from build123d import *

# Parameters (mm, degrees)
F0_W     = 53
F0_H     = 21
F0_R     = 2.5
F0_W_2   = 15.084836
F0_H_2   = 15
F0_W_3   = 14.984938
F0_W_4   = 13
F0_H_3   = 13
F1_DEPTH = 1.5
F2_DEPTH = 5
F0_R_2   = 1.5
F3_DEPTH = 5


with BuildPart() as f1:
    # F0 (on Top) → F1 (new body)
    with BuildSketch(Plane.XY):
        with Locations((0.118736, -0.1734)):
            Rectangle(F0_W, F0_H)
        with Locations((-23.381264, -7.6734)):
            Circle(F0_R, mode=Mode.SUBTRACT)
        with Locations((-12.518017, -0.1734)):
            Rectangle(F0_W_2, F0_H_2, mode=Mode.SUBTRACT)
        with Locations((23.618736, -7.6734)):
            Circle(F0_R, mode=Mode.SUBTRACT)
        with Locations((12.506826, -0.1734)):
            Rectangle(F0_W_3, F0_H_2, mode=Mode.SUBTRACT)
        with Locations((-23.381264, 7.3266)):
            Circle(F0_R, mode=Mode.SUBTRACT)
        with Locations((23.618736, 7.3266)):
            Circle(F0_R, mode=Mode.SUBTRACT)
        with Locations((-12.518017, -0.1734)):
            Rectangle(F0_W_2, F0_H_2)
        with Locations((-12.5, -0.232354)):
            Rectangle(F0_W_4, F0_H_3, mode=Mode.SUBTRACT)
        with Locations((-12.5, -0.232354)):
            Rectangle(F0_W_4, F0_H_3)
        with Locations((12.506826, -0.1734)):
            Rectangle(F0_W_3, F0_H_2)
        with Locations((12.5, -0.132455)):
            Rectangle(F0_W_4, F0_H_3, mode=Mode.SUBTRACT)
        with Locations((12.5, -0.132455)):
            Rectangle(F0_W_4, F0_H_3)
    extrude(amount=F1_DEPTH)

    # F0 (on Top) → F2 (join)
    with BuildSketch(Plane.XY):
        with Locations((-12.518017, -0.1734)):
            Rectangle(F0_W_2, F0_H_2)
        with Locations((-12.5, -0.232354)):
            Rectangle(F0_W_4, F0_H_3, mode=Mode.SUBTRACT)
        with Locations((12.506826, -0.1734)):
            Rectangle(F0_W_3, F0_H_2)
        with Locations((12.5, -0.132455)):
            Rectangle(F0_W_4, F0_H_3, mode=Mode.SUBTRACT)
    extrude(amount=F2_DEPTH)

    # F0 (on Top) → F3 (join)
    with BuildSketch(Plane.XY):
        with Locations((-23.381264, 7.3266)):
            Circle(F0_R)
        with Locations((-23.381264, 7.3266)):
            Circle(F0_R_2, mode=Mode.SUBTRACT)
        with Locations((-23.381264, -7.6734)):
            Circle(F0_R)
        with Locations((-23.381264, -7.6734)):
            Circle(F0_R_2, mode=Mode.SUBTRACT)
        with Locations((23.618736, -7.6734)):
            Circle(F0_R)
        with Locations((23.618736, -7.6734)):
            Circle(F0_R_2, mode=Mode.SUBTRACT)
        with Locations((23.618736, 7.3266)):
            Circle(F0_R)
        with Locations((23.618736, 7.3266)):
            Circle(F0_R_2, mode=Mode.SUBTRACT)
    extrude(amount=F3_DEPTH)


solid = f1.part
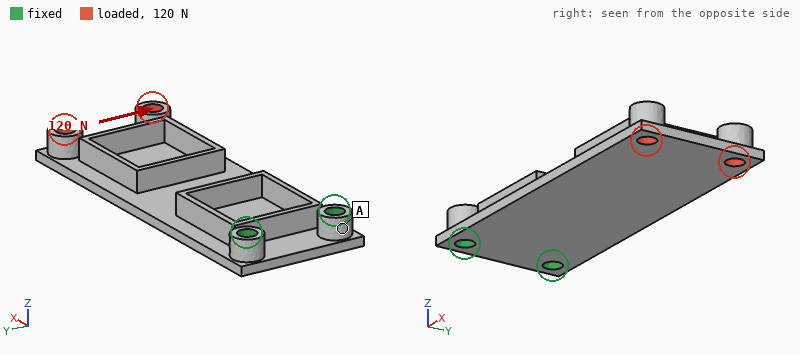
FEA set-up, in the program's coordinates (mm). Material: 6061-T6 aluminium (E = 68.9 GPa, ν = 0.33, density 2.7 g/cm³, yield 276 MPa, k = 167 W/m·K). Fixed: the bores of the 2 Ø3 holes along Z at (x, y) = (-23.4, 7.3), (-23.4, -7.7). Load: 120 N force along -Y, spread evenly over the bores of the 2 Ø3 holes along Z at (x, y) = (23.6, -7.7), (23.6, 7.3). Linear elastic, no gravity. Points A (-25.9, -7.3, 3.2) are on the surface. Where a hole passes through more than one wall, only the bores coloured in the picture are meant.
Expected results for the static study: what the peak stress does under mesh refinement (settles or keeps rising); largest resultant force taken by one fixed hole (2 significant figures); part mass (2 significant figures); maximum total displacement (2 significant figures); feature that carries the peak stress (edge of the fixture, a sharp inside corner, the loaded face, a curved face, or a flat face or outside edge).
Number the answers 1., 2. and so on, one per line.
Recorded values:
1. keeps rising
2. 360 N
3. 5.9 g
4. 0.15 mm
5. edge of the fixture
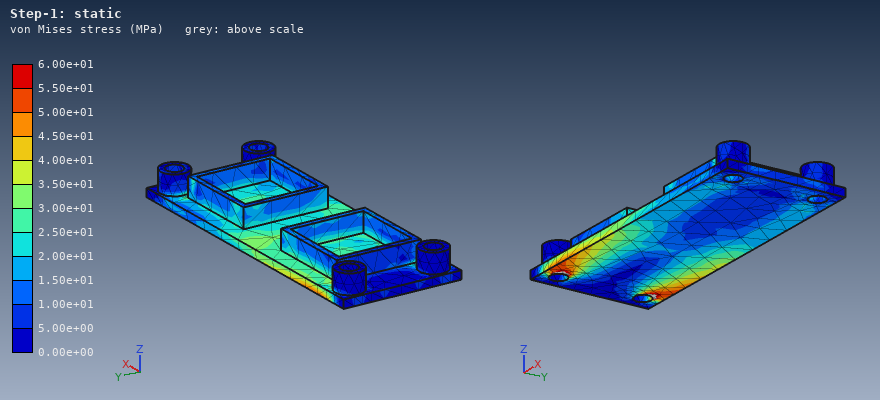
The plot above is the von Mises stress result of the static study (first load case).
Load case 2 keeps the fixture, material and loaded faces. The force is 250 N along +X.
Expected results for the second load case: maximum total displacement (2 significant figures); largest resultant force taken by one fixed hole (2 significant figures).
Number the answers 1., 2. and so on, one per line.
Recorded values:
1. 0.62 mm
2. 130 N
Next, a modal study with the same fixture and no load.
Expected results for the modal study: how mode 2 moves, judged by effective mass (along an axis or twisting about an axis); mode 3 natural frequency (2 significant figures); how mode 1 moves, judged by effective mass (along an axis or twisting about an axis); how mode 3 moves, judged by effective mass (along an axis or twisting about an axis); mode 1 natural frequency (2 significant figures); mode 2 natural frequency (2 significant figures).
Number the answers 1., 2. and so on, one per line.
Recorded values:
1. twisting about X
2. 3400 Hz
3. along Z
4. along Z
5. 620 Hz
6. 2400 Hz
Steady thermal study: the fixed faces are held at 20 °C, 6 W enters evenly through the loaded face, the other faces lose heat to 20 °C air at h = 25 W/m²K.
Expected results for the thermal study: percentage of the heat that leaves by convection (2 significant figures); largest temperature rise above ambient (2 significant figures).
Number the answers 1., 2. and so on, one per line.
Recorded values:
1. 26 %
2. 42 K
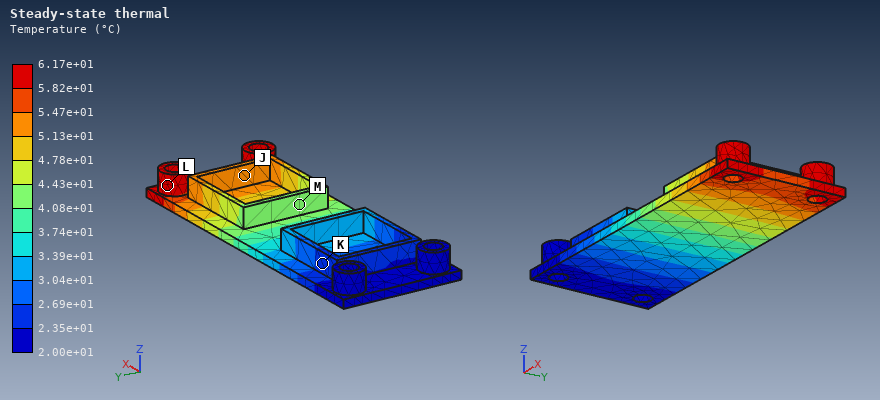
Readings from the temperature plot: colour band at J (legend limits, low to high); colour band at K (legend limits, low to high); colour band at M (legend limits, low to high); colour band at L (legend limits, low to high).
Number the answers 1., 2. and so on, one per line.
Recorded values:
1. 5.13e+01 to 5.47e+01 °C
2. 2.35e+01 to 2.69e+01 °C
3. 4.08e+01 to 4.43e+01 °C
4. 5.82e+01 to 6.17e+01 °C
